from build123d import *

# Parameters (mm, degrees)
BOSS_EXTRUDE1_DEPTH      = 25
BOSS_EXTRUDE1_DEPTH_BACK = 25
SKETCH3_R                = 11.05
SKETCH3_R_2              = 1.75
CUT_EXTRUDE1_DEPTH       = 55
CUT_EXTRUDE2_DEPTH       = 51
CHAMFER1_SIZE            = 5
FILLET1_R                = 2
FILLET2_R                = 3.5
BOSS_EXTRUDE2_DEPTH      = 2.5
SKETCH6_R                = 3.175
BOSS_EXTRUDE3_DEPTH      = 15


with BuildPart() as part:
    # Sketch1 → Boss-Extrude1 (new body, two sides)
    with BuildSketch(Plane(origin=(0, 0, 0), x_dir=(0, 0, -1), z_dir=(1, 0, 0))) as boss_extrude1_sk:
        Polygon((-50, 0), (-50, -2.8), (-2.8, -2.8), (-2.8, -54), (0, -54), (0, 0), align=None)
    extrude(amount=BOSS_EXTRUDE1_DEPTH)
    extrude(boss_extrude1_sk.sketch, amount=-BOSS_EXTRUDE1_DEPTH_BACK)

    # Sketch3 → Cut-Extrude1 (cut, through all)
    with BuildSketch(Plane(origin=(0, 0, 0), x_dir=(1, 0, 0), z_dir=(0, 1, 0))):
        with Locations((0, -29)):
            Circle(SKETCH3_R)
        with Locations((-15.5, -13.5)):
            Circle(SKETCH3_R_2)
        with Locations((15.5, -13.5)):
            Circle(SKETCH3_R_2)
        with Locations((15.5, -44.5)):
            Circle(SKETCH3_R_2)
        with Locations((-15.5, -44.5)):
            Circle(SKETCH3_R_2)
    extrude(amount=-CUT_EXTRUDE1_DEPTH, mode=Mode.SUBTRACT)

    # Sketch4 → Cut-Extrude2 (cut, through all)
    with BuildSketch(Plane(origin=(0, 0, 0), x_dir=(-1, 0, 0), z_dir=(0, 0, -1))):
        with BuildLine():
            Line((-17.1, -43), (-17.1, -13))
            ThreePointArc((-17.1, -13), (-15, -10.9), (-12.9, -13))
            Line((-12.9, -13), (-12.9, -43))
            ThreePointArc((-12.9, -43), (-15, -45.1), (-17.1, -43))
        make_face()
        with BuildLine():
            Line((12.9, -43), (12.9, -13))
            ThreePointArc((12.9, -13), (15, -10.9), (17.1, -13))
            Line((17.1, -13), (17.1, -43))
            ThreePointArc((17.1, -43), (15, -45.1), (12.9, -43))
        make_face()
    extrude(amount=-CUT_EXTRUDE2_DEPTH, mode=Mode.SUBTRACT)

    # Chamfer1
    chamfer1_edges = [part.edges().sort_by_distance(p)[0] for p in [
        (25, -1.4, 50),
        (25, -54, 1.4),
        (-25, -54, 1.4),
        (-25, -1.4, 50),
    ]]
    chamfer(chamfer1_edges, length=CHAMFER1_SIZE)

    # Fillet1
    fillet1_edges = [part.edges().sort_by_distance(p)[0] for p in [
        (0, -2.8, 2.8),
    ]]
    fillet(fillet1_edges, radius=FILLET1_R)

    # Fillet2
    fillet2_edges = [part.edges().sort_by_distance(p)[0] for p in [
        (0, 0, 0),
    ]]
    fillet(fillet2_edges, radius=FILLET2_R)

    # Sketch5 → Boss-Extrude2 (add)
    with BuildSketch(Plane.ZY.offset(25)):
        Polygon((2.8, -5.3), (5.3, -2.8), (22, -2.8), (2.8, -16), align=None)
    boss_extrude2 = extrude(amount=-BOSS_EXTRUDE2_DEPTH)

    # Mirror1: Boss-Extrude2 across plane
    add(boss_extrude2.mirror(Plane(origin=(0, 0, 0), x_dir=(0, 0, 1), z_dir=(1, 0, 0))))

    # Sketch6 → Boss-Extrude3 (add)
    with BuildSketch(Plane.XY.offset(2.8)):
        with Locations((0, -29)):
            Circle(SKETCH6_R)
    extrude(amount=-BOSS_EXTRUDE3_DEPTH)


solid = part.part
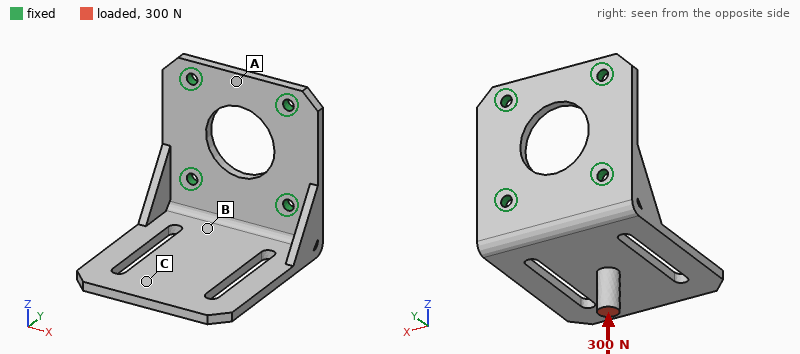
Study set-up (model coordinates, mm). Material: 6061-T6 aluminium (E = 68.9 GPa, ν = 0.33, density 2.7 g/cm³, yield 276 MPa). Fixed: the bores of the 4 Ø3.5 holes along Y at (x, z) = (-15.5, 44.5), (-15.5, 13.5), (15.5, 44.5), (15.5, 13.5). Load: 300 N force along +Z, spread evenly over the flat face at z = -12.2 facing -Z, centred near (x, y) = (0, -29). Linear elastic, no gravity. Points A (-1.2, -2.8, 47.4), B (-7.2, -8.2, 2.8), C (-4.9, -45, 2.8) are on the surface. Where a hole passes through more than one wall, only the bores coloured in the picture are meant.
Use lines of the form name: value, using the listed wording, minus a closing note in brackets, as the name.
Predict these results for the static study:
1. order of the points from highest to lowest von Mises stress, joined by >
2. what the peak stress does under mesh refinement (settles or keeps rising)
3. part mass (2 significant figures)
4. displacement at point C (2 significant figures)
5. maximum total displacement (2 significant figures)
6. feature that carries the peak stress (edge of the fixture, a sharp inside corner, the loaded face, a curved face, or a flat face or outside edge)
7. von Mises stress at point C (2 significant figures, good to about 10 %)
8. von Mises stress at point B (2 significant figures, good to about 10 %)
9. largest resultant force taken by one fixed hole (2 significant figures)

order of the points from highest to lowest von Mises stress, joined by >: B > C > A
what the peak stress does under mesh refinement: keeps rising
part mass: 35 g
displacement at point C: 0.72 mm
maximum total displacement: 0.90 mm
feature that carries the peak stress: edge of the fixture
von Mises stress at point C: 29 MPa
von Mises stress at point B: 70 MPa
largest resultant force taken by one fixed hole: 180 N
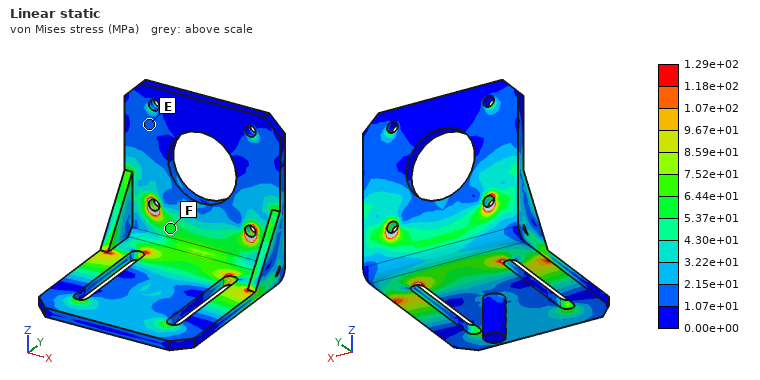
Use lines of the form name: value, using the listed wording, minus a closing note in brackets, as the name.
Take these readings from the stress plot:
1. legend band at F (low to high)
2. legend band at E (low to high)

legend band at F: 5.37e+01 to 6.44e+01 MPa
legend band at E: 1.07e+01 to 2.15e+01 MPa
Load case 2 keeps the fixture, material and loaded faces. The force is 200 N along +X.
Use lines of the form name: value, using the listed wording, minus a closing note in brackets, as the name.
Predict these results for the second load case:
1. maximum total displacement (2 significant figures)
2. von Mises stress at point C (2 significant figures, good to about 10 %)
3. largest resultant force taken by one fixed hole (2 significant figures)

maximum total displacement: 0.13 mm
von Mises stress at point C: 9.9 MPa
largest resultant force taken by one fixed hole: 220 N
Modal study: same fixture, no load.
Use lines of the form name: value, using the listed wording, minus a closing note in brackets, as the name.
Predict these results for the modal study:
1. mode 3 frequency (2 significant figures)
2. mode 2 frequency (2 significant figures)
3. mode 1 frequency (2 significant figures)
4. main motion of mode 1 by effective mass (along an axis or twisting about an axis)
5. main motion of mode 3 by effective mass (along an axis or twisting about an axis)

mode 3 frequency: 3000 Hz
mode 2 frequency: 2100 Hz
mode 1 frequency: 840 Hz
main motion of mode 1 by effective mass: along Z
main motion of mode 3 by effective mass: along X
